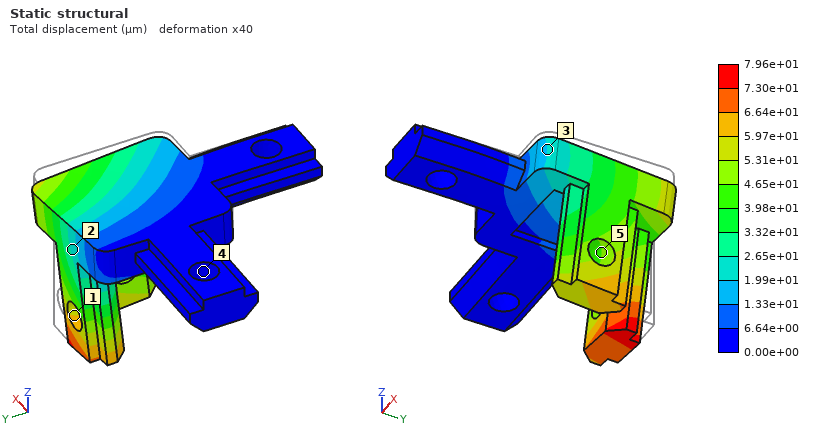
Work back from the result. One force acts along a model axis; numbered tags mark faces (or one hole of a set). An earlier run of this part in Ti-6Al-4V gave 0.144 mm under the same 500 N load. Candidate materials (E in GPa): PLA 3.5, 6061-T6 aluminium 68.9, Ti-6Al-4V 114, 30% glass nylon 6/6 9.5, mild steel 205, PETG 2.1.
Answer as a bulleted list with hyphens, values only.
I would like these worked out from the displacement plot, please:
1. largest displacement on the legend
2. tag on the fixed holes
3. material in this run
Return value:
- 7.96e+01 µm
- 4
- mild steel
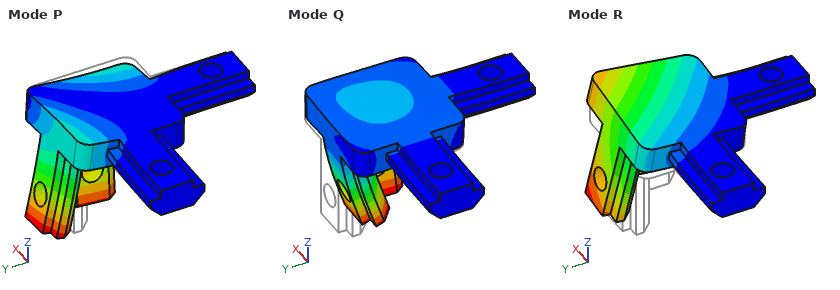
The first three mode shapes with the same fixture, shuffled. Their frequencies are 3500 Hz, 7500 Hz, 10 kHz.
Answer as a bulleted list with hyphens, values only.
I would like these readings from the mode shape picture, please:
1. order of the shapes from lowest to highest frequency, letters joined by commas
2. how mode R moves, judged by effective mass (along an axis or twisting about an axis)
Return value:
- R, P, Q
- along Z
